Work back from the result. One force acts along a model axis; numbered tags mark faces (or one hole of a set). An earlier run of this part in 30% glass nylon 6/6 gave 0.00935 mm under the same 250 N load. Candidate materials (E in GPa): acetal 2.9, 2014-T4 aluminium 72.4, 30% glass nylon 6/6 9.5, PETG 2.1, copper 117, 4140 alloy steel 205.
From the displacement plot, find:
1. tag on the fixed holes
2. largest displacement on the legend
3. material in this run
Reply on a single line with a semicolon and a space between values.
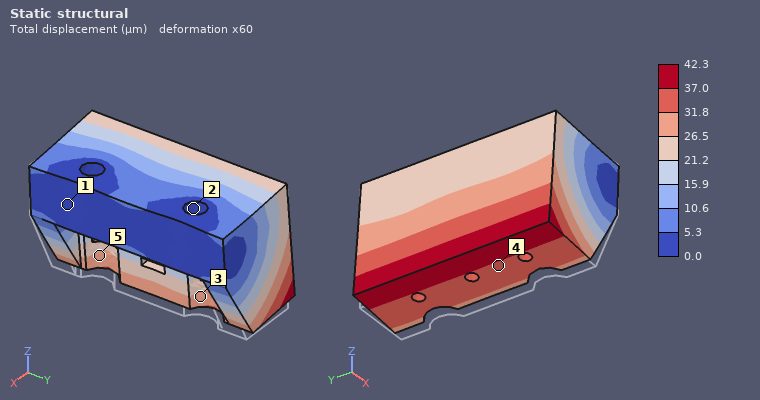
2; 42.3 µm; PETG
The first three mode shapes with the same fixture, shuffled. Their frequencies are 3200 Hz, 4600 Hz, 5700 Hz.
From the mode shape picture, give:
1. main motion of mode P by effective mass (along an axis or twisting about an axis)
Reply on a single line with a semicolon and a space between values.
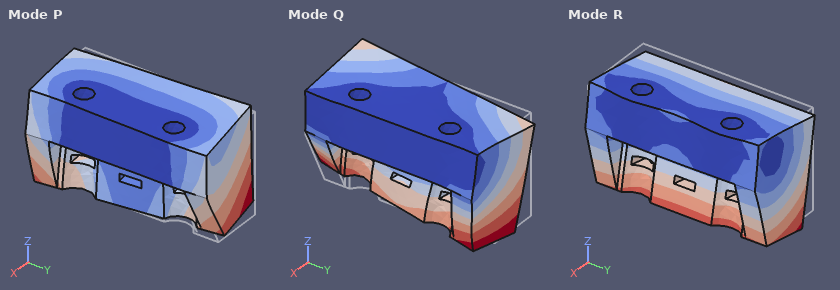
along Y
